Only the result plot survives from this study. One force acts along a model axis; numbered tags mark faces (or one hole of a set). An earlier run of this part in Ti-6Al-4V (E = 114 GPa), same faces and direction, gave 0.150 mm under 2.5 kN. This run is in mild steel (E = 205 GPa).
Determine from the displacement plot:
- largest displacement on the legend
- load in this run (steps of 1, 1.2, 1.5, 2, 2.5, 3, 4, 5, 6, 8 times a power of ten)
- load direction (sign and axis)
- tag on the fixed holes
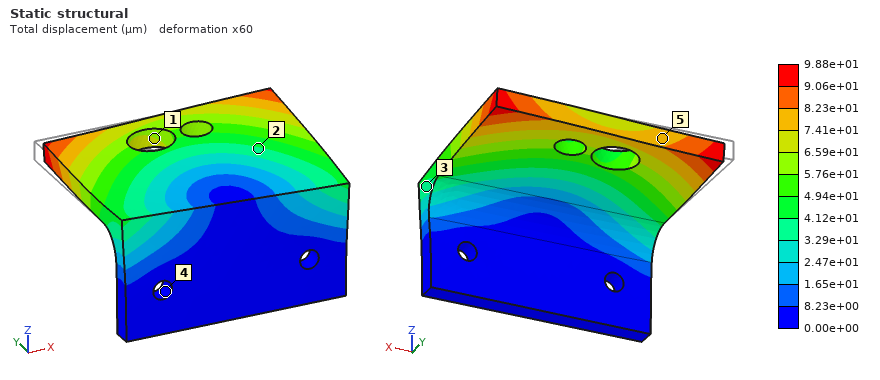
9.88e+01 µm
3 kN
+X
4
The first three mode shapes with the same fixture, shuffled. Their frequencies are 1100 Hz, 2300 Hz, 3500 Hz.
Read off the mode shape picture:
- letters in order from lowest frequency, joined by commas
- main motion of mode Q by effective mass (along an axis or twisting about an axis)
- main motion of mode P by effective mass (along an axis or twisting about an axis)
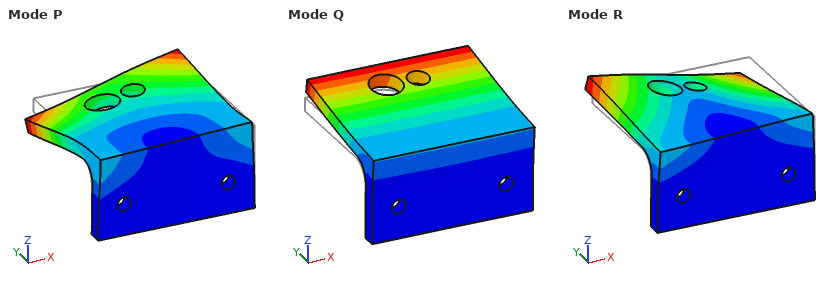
Q, R, P
along Z
along X
